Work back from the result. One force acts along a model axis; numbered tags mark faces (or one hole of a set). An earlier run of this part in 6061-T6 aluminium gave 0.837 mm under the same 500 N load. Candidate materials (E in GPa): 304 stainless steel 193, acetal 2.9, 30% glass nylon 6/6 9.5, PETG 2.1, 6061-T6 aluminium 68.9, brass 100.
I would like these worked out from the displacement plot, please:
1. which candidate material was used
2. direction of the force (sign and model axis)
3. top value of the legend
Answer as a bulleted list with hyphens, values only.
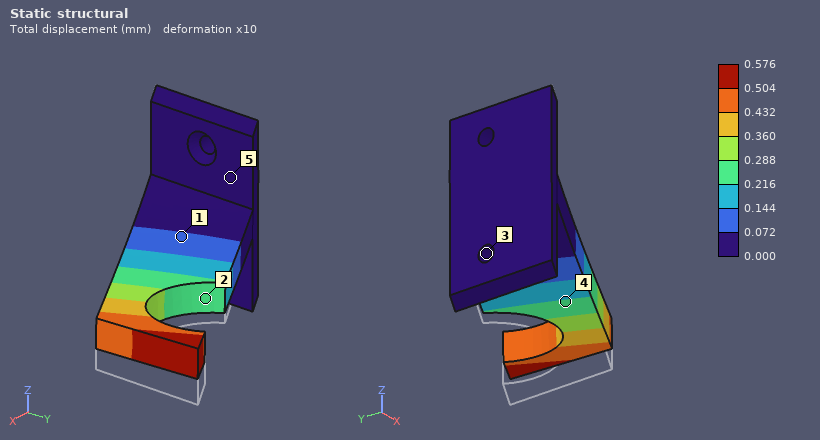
- brass
- +Z
- 0.576 mm
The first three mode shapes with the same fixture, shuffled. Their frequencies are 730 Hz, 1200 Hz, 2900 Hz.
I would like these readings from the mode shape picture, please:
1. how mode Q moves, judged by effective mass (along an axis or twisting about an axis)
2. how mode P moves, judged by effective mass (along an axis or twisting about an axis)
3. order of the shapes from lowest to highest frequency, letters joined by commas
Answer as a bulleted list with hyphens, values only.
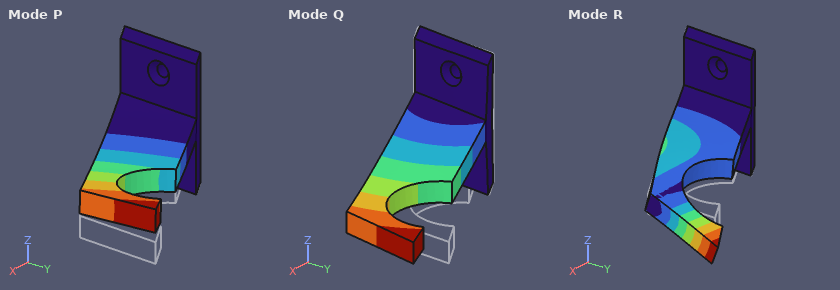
- along Y
- along Z
- P, Q, R
